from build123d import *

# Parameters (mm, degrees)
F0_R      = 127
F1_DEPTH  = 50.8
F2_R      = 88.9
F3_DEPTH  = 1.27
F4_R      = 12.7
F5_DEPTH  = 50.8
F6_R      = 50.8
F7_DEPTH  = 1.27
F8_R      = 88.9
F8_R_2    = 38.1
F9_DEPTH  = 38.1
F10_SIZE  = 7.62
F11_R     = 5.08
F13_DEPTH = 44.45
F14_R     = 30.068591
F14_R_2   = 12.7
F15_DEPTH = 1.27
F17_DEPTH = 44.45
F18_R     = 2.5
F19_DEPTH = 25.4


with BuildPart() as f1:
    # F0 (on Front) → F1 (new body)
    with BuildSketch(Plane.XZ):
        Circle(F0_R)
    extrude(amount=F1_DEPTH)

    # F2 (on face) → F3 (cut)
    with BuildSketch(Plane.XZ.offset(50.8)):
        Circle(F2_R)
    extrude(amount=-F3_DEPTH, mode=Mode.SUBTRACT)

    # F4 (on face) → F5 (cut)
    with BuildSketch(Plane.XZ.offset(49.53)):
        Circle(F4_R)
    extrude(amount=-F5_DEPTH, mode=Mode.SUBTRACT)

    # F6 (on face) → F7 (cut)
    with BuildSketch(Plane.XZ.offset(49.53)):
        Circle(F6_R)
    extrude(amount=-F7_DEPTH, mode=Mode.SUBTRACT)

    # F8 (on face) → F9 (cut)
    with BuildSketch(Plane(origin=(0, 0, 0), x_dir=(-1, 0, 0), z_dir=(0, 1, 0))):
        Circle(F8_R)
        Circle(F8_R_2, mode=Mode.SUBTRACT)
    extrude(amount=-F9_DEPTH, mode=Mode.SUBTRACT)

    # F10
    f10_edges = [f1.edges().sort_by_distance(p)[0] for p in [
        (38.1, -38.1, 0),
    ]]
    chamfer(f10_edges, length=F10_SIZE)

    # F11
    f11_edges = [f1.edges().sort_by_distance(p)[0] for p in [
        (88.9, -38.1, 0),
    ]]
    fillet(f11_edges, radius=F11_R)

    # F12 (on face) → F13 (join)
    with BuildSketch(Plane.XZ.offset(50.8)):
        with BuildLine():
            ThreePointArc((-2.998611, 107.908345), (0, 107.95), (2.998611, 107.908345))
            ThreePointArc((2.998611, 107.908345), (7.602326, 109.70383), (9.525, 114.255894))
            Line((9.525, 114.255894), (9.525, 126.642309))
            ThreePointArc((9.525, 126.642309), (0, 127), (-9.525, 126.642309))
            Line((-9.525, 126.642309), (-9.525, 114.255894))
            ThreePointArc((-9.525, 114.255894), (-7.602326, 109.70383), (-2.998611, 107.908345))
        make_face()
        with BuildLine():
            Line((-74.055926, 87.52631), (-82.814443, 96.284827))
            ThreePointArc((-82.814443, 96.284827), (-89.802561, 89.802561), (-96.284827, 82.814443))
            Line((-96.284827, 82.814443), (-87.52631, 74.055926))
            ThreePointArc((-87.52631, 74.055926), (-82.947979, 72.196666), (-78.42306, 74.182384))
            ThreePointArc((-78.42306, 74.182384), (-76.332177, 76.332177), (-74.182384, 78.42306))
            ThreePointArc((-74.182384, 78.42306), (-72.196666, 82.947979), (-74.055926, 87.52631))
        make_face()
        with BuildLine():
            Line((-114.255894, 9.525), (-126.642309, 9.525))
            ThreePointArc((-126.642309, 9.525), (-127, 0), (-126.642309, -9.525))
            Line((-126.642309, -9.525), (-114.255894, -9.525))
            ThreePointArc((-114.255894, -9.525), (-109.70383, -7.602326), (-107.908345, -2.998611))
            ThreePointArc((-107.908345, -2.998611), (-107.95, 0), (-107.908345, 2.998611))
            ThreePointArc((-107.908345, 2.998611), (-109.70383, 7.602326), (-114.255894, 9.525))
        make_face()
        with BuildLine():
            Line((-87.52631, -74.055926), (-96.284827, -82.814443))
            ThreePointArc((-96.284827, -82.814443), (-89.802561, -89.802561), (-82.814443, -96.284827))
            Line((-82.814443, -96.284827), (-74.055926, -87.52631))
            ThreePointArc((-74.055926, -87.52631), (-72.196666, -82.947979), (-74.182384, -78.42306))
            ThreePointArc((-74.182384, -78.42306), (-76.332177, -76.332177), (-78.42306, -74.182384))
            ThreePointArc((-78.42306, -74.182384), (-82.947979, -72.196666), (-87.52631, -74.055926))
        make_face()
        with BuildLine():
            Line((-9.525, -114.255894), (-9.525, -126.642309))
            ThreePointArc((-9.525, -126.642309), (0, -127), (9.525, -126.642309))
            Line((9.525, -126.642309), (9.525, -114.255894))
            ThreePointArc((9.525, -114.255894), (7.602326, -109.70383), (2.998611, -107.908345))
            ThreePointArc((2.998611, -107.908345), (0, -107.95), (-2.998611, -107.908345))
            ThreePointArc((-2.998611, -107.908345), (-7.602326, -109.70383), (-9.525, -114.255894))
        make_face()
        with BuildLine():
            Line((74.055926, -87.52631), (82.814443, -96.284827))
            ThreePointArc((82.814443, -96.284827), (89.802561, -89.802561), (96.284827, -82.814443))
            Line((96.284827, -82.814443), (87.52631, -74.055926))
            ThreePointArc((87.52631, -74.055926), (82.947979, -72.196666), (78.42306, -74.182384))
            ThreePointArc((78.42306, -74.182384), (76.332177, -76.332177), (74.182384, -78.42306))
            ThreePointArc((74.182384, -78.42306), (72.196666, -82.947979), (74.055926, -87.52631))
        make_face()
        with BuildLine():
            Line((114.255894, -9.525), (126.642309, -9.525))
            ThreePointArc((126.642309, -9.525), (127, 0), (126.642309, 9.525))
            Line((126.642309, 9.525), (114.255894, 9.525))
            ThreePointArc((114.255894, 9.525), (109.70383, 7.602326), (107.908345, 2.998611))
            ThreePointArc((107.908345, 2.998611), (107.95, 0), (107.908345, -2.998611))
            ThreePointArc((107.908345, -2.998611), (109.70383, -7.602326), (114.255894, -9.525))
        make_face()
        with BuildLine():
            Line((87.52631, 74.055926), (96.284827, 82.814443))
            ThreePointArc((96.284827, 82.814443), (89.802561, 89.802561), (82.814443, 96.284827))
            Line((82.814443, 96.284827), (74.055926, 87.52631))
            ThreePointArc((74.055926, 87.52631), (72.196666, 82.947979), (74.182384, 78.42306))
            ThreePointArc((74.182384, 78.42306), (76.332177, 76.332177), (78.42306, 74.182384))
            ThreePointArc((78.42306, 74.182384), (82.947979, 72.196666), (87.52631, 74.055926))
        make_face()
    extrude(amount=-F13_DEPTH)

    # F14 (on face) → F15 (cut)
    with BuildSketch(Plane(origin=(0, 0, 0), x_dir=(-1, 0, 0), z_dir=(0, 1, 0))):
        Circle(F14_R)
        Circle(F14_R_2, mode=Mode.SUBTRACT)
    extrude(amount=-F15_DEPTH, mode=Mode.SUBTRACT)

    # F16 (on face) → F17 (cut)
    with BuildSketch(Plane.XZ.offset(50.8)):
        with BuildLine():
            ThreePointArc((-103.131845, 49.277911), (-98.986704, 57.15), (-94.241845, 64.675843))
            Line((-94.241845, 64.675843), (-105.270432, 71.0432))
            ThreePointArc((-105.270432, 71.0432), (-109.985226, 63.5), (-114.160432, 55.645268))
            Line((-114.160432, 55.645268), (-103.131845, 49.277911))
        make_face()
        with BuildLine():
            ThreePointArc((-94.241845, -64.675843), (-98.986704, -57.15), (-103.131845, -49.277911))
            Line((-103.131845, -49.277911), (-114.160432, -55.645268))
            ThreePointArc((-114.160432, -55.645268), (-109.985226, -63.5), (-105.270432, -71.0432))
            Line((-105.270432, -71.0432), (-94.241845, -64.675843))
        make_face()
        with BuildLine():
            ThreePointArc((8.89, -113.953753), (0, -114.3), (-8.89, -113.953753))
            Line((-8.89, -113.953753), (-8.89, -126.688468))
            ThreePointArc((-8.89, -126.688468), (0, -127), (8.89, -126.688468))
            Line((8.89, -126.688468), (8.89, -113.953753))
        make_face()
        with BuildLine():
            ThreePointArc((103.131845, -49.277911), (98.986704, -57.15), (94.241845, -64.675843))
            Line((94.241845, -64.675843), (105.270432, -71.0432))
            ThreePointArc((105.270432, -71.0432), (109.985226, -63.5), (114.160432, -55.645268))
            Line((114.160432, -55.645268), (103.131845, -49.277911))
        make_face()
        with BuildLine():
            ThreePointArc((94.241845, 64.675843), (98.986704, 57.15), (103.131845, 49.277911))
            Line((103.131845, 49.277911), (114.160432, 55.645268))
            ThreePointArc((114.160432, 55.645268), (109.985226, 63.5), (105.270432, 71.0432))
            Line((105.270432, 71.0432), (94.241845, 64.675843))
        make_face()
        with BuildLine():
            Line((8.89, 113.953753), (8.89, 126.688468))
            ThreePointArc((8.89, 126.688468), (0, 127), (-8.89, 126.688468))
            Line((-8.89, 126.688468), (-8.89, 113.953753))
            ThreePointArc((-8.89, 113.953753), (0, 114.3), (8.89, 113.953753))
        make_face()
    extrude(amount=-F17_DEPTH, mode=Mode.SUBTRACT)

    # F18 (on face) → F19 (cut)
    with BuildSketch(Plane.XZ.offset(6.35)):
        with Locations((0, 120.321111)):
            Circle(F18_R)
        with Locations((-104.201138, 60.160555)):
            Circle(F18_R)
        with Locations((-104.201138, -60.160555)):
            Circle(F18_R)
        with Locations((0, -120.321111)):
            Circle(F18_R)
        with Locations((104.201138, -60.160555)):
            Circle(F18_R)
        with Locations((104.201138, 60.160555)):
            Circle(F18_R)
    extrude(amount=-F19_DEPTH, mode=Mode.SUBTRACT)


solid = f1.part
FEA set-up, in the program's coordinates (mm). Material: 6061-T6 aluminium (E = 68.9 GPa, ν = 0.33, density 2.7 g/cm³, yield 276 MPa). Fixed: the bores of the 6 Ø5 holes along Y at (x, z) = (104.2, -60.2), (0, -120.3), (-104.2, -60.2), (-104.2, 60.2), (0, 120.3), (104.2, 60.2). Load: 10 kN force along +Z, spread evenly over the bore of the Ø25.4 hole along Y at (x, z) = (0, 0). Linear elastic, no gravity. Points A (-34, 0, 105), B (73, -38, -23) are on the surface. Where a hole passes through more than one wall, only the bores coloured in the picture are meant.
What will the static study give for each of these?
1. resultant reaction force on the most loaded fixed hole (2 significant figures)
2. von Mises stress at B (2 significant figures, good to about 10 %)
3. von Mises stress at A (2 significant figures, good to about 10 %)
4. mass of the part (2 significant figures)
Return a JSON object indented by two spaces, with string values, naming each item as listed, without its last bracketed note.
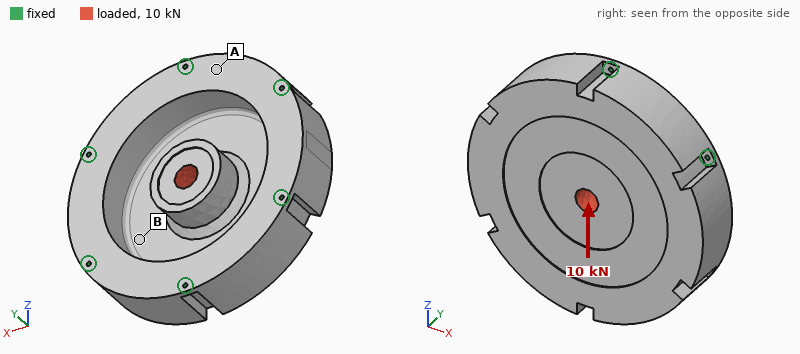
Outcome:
{
  "resultant reaction force on the most loaded fixed hole": "2.2 kN",
  "von Mises stress at B": "5.7 MPa",
  "von Mises stress at A": "2.0 MPa",
  "mass of the part": "4.5 kg"
}
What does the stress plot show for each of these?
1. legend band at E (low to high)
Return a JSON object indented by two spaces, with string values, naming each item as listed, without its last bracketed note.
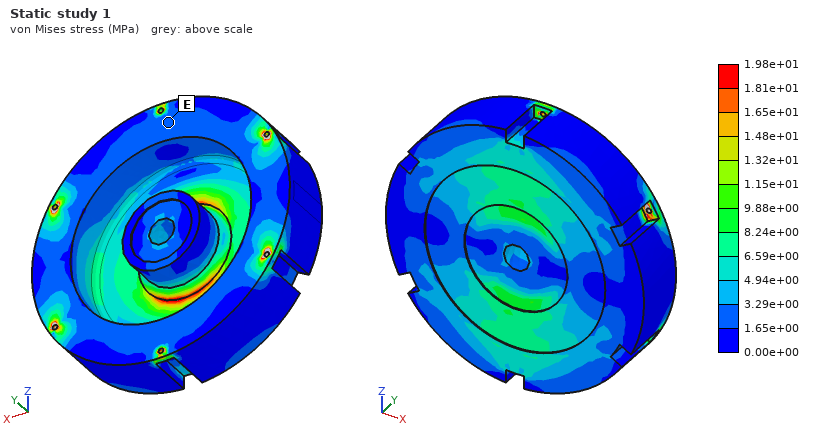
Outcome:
{
  "legend band at E": "1.65e+00 to 3.29e+00 MPa"
}
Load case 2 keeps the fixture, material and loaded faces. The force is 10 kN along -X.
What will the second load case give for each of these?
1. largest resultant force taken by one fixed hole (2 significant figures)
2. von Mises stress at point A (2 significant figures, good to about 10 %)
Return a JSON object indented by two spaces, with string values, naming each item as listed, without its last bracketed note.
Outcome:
{
  "largest resultant force taken by one fixed hole": "2.5 kN",
  "von Mises stress at point A": "2.6 MPa"
}
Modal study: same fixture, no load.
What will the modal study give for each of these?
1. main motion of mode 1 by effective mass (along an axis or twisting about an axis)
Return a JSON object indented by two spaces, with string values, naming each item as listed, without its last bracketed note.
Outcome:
{
  "main motion of mode 1 by effective mass": "along Y"
}
